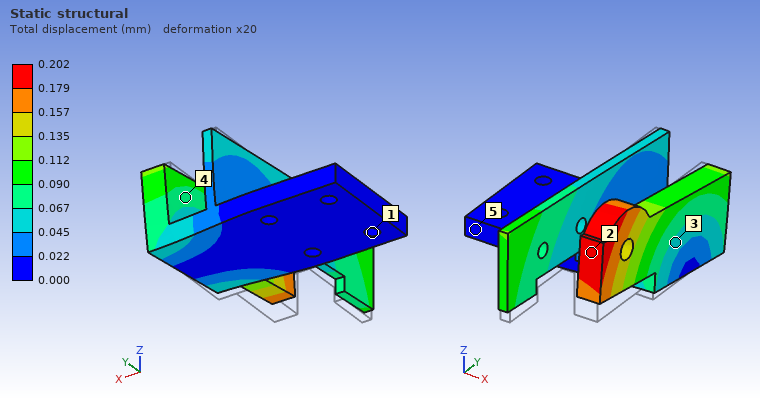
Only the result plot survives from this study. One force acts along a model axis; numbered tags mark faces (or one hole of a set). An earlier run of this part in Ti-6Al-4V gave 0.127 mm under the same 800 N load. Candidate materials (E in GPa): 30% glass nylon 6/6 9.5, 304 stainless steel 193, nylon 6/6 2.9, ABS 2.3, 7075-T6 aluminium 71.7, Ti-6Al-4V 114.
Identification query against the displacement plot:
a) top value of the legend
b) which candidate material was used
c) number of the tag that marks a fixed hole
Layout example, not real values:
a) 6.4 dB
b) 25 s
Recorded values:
a) 0.202 mm
b) 7075-T6 aluminium
c) 1
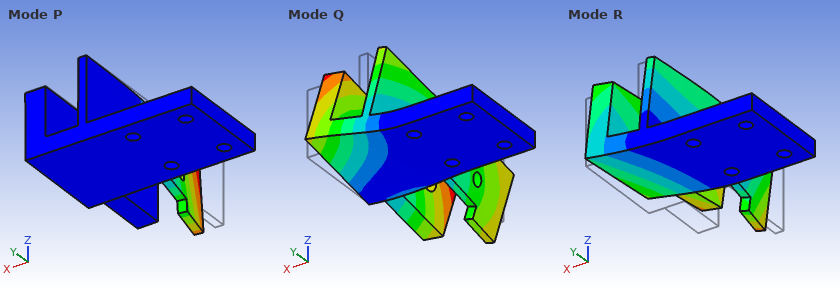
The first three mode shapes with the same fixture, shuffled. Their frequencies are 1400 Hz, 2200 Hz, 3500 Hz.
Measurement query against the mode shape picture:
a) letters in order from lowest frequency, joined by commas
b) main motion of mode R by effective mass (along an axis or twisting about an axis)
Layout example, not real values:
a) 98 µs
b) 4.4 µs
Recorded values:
a) P, R, Q
b) along Z
